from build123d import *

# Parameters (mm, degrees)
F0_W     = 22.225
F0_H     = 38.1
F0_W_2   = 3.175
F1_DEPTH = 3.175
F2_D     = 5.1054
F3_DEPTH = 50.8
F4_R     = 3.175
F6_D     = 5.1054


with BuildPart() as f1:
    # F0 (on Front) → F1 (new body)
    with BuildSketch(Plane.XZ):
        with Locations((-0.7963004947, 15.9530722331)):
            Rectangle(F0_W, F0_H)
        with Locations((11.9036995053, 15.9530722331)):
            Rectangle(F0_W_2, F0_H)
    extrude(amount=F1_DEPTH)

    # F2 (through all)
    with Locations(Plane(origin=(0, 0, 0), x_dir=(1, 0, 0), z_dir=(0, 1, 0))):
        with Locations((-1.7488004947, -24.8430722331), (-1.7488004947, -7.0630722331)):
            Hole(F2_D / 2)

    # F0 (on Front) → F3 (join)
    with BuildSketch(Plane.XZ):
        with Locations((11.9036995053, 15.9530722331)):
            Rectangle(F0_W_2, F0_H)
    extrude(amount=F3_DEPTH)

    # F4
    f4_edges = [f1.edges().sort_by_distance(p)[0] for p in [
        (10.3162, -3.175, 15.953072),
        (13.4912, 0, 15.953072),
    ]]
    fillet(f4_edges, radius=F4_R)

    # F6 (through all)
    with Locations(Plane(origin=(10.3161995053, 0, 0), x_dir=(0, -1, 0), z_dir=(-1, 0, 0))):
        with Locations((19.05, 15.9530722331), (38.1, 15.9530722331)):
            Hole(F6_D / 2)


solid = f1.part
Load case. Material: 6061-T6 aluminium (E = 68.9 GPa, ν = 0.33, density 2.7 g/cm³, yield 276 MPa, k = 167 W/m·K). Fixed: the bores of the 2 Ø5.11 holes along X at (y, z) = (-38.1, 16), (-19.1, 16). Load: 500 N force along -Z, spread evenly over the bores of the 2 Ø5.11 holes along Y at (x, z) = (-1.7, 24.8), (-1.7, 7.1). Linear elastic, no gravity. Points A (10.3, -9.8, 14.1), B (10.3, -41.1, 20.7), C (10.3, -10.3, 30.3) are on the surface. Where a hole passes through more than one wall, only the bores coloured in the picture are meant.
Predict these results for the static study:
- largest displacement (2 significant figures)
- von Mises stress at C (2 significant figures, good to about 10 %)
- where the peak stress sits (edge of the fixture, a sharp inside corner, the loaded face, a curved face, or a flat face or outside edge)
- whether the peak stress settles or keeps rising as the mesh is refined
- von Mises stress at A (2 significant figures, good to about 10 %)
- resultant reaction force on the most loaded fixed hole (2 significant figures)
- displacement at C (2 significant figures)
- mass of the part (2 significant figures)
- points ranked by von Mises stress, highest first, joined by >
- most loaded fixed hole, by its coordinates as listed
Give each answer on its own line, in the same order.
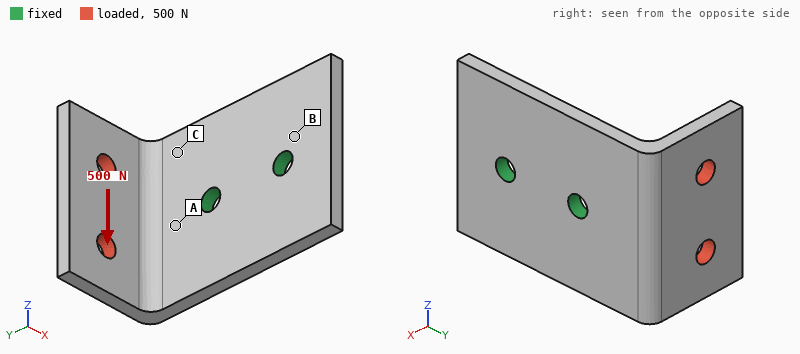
0.28 mm
44 MPa
edge of the fixture
keeps rising
79 MPa
830 N
0.088 mm
23 g
A > C > B
(-19.1, 16)
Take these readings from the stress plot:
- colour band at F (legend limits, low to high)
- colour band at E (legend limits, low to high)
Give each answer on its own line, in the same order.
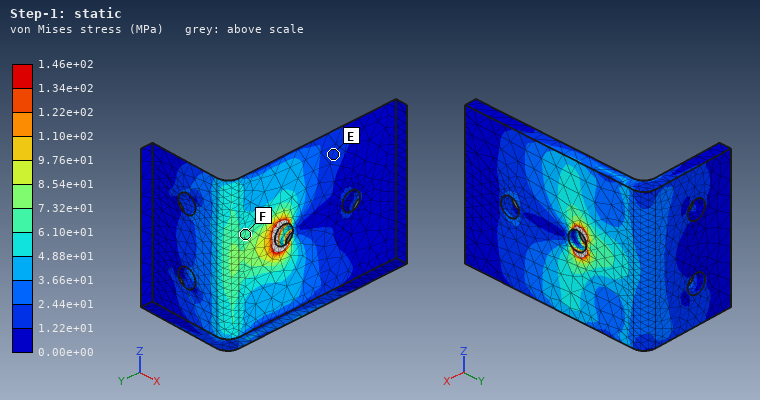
6.10e+01 to 7.32e+01 MPa
1.22e+01 to 2.44e+01 MPa
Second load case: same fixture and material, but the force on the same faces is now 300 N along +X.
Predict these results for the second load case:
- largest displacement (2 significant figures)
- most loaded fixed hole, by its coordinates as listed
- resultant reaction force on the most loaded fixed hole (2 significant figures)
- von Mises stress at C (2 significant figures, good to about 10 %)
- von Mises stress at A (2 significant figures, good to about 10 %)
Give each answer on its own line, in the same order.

0.18 mm
(-19.1, 16)
390 N
33 MPa
42 MPa
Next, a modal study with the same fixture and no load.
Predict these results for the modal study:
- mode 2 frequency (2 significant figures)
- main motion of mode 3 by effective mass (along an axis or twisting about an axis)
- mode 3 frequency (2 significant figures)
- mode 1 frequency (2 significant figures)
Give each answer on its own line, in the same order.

2700 Hz
along X
5900 Hz
2100 Hz
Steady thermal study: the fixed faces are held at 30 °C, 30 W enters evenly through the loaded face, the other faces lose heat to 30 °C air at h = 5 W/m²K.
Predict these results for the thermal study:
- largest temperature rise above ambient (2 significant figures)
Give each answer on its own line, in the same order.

52 K
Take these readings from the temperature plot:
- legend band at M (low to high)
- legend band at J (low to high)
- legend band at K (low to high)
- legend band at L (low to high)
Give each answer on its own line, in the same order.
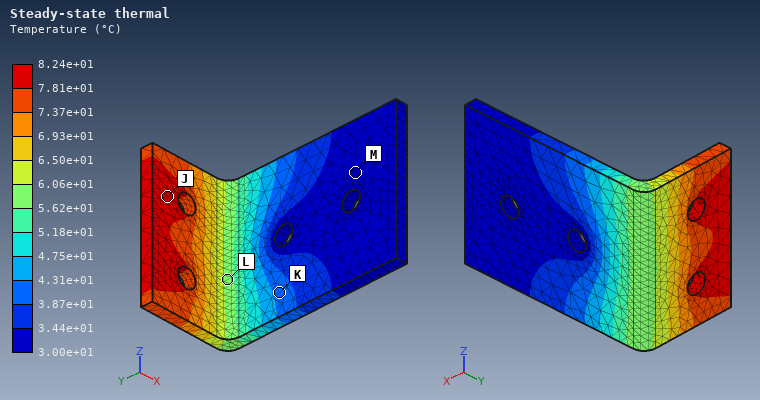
3.00e+01 to 3.44e+01 °C
7.81e+01 to 8.24e+01 °C
3.87e+01 to 4.31e+01 °C
5.62e+01 to 6.06e+01 °C
